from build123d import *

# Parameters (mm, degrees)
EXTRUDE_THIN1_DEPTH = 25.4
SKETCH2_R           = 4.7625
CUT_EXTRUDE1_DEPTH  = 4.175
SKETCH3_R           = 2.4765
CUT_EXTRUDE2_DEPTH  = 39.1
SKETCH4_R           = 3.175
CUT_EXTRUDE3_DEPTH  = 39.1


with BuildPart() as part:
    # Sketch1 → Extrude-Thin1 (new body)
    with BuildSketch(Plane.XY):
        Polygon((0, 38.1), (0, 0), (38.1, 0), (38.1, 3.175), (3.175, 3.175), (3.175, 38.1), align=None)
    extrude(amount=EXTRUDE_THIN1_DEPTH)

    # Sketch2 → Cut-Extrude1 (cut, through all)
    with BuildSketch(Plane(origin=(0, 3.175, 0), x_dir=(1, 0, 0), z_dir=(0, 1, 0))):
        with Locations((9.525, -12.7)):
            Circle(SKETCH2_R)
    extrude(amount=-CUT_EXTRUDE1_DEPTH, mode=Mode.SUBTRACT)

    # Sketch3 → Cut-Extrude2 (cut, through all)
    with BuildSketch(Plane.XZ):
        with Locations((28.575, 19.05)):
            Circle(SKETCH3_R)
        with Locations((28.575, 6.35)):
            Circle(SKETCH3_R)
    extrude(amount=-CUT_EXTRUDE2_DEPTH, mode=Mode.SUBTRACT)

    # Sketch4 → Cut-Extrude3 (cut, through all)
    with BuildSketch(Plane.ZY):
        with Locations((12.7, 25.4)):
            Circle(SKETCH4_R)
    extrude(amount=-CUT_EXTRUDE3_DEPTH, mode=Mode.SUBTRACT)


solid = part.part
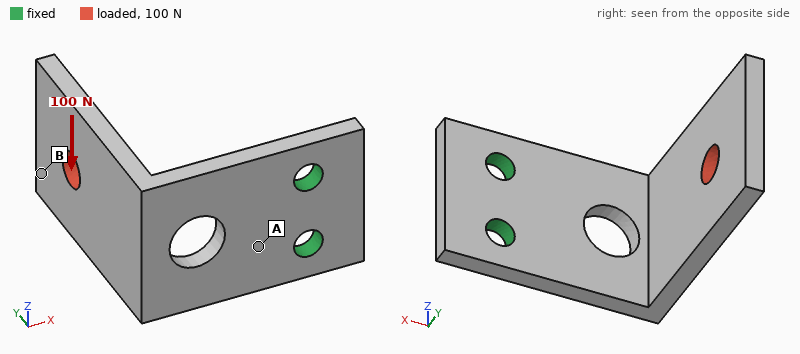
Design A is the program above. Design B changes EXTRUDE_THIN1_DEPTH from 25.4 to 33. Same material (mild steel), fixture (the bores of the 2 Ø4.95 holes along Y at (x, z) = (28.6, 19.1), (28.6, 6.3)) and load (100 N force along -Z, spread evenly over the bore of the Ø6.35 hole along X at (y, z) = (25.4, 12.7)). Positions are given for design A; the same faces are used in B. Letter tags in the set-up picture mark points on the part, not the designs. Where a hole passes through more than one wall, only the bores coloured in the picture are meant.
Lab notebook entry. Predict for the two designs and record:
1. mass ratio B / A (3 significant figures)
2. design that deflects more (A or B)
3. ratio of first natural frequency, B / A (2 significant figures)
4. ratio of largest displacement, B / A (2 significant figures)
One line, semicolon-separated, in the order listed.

1.32; A; 1.0; 0.75
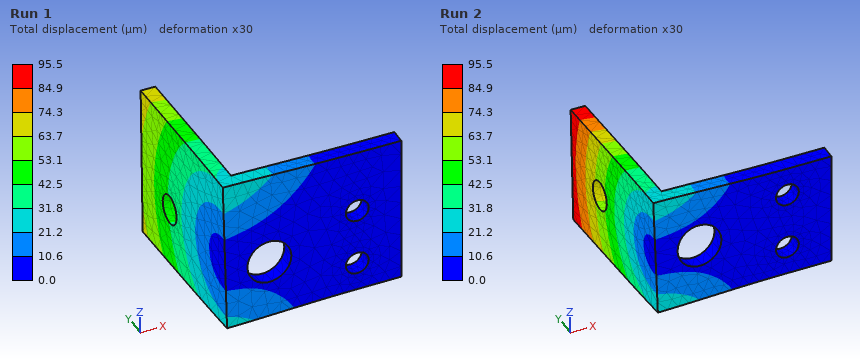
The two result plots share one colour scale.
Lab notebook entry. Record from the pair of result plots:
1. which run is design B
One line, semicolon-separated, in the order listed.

Run 1
